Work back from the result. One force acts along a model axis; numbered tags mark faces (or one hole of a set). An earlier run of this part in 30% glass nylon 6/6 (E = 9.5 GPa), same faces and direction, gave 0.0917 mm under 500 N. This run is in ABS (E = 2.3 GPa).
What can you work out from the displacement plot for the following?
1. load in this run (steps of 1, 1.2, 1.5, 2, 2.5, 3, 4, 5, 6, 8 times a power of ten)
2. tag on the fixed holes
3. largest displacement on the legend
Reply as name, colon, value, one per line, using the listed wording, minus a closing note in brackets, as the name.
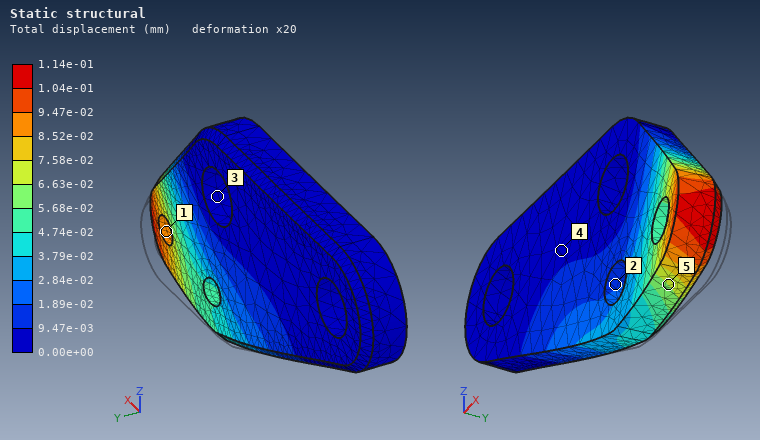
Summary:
load in this run: 150 N
tag on the fixed holes: 3
largest displacement on the legend: 1.14e-01 mm
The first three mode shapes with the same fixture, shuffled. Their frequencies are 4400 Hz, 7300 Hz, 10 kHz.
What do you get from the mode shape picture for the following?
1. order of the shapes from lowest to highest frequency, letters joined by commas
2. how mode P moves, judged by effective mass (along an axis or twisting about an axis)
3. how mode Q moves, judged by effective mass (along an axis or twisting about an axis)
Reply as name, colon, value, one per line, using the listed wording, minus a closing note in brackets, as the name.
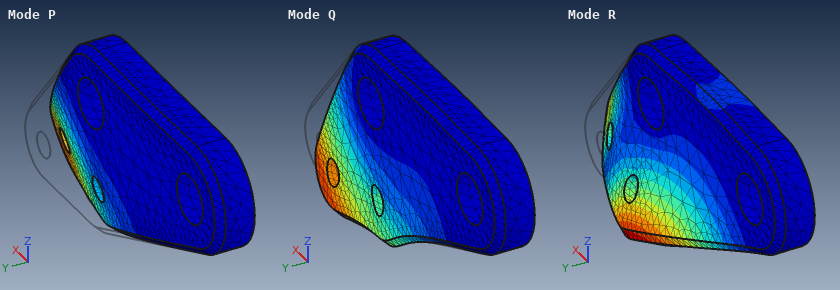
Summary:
order of the shapes from lowest to highest frequency, letters joined by commas: P, R, Q
how mode P moves, judged by effective mass: along Y
how mode Q moves, judged by effective mass: along X
